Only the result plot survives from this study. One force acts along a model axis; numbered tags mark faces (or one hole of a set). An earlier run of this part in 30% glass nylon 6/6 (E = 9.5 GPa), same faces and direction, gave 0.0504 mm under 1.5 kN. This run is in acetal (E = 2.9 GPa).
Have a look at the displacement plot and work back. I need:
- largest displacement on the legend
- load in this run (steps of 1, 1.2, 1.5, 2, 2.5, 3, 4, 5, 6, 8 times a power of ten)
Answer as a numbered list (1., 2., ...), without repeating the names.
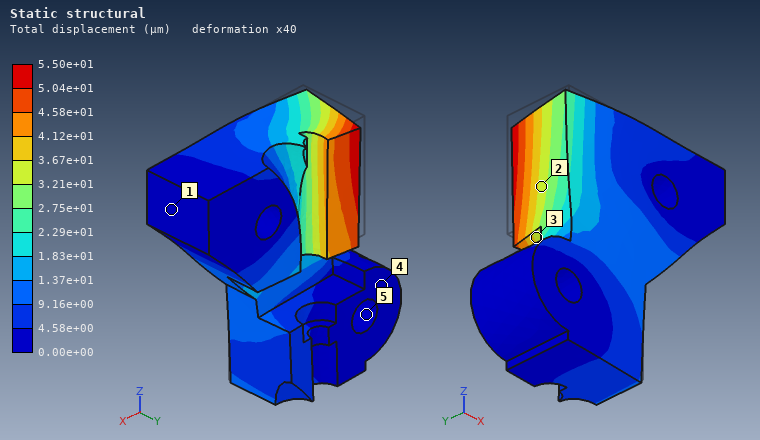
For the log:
1. 5.50e+01 µm
2. 500 N
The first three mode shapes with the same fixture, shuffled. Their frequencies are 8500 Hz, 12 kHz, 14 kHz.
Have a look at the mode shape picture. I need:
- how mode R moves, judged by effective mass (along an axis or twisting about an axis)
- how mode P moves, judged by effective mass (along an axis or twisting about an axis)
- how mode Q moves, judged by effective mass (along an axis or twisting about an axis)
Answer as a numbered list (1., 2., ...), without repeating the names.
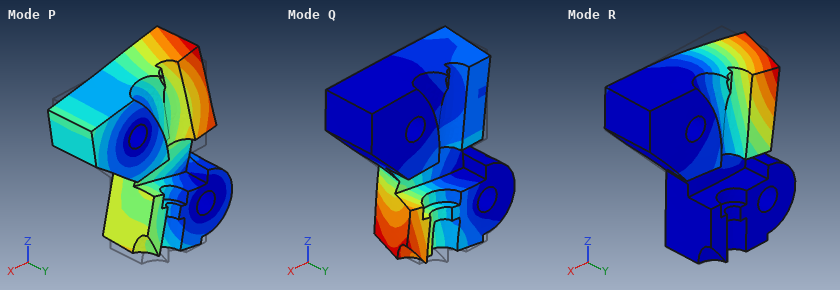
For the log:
1. along Y
2. along Z
3. along Y
